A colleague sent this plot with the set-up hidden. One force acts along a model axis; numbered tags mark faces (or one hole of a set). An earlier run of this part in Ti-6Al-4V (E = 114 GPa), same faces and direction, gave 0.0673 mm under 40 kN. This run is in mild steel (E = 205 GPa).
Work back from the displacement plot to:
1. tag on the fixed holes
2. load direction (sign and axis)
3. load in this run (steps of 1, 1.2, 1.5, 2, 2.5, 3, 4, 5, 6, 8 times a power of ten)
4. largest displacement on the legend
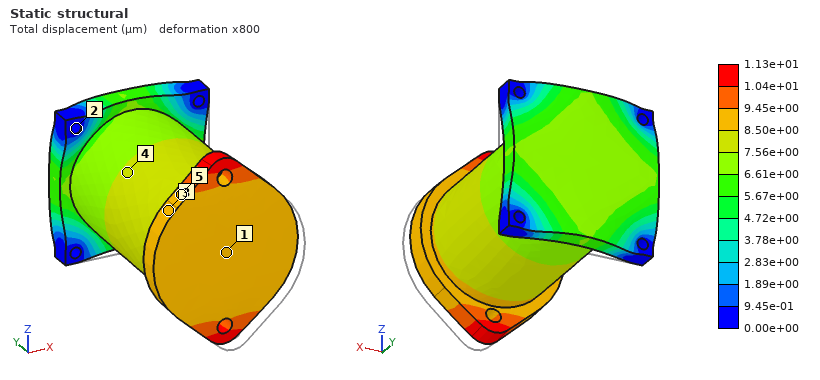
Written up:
2
+Y
12 kN
1.13e+01 µm
